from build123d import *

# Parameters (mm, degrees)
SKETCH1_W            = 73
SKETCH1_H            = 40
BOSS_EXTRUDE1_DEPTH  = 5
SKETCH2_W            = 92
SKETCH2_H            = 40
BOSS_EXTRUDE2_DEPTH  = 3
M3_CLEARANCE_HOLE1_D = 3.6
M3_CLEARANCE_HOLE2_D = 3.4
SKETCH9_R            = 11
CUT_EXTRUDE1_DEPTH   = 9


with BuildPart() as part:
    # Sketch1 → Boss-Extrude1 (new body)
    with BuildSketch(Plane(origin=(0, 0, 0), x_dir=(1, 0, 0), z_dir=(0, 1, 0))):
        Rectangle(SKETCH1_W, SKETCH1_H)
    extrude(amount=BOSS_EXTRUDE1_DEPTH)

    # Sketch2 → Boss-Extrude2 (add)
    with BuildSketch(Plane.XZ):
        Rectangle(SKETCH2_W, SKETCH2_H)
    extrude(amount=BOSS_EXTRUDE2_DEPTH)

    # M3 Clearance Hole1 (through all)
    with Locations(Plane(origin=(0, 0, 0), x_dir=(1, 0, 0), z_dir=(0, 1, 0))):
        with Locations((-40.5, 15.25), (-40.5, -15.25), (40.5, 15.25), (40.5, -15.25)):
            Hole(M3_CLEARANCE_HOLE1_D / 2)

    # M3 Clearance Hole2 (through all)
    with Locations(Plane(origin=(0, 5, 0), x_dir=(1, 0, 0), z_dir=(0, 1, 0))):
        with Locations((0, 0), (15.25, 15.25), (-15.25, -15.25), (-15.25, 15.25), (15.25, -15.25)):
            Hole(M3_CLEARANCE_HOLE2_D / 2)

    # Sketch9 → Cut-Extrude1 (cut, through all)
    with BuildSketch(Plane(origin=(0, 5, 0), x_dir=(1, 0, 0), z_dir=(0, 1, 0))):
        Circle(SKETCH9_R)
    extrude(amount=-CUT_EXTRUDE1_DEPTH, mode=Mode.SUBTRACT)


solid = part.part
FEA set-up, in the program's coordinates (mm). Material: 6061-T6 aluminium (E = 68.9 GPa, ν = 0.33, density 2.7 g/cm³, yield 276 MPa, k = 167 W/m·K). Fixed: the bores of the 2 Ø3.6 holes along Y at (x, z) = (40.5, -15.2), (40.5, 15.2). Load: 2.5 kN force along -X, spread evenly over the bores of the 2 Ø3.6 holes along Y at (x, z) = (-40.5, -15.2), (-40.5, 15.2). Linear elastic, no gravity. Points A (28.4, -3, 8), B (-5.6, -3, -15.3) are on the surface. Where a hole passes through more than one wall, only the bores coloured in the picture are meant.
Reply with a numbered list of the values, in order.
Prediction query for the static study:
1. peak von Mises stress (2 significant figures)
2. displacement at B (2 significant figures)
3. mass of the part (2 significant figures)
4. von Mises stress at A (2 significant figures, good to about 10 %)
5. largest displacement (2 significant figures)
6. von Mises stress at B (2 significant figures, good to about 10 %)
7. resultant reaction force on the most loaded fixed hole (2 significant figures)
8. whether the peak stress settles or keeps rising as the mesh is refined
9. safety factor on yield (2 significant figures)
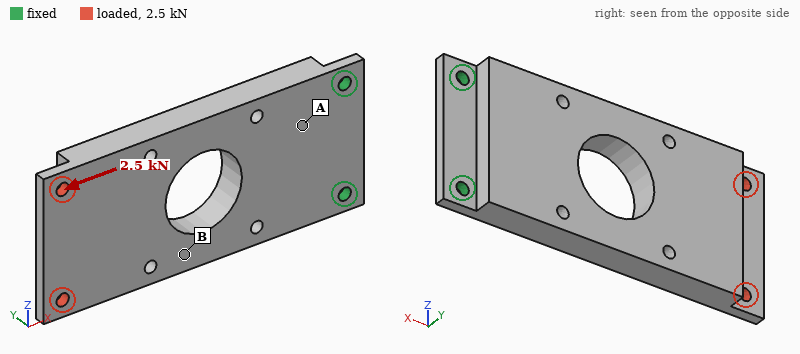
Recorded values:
1. 97 MPa
2. 0.067 mm
3. 60 g
4. 19 MPa
5. 0.27 mm
6. 43 MPa
7. 1.3 kN
8. settles
9. 2.9
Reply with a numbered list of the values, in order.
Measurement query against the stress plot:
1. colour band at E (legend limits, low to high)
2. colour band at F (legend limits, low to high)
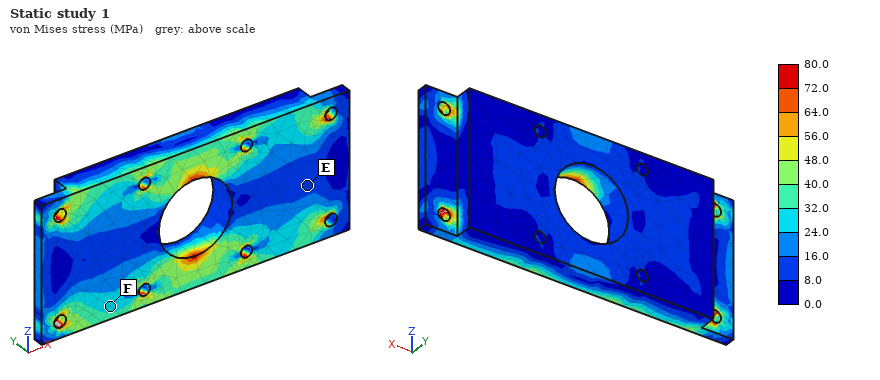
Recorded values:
1. 8.0 to 16.0 MPa
2. 24.0 to 32.0 MPa
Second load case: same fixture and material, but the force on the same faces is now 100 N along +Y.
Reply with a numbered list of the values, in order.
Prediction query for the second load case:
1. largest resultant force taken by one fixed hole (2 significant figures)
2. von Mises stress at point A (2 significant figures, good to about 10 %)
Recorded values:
1. 84 N
2. 18 MPa
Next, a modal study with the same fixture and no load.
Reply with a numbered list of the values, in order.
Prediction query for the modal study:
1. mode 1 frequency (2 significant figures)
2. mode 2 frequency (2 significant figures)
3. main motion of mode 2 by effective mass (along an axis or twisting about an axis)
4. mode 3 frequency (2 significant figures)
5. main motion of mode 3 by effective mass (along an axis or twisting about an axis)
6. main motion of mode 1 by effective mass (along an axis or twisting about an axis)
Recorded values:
1. 420 Hz
2. 2800 Hz
3. along Z
4. 3400 Hz
5. along Z
6. along Y
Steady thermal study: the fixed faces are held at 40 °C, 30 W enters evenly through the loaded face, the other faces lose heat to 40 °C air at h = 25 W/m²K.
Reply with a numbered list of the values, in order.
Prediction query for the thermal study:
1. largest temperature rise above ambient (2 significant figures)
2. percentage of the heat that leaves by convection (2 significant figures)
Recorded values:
1. 73 K
2. 25 %
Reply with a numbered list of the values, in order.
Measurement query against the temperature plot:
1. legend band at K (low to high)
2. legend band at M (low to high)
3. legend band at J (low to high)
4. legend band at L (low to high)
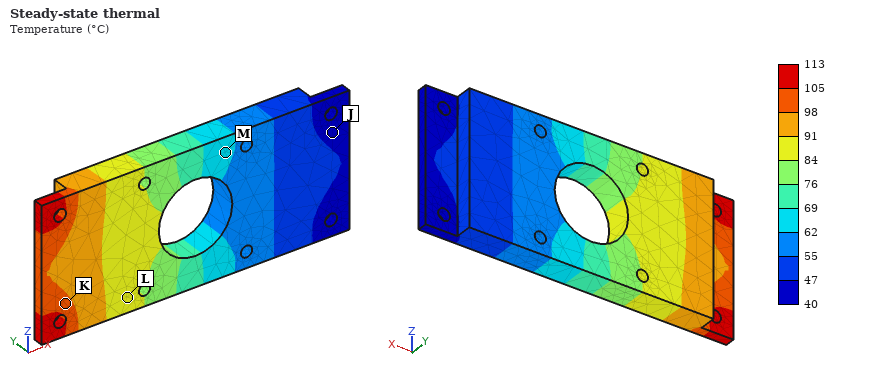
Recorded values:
1. 98 to 105 °C
2. 62 to 69 °C
3. 40 to 47 °C
4. 84 to 91 °C
